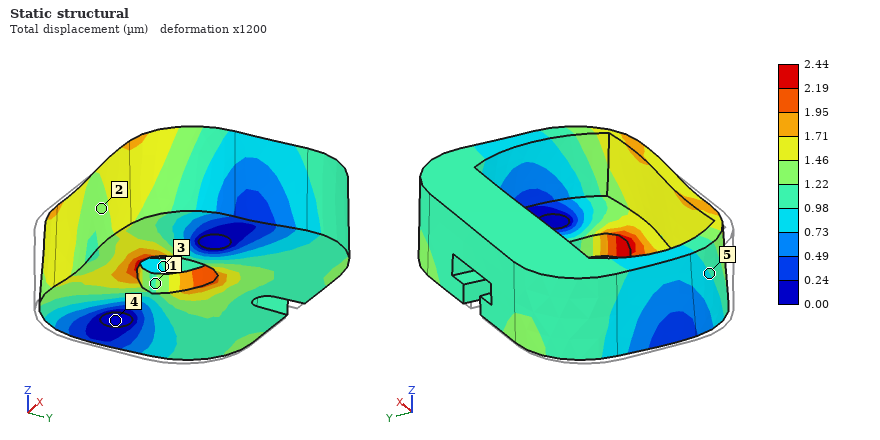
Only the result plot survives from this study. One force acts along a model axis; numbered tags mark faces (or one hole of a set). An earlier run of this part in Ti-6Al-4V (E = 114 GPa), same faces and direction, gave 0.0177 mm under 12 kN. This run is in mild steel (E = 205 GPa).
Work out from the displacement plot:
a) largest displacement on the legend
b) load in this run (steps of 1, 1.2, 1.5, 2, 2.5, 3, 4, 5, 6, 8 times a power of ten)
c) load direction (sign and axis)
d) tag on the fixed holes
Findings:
2.44 µm
3 kN
+X
4
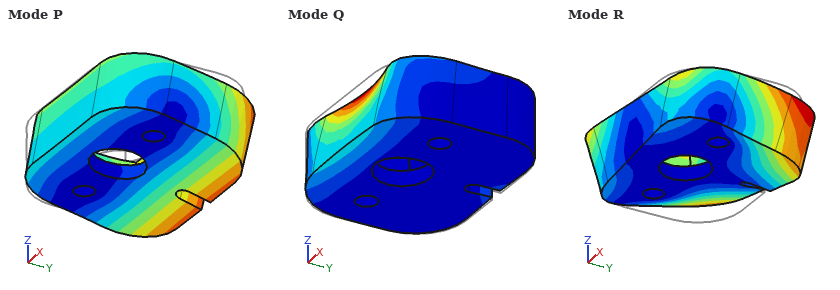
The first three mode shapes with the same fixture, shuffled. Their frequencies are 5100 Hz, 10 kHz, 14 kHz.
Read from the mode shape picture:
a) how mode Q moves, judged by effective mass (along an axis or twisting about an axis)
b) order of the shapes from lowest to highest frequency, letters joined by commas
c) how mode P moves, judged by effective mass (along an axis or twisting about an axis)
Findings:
along Z
P, R, Q
along Z
